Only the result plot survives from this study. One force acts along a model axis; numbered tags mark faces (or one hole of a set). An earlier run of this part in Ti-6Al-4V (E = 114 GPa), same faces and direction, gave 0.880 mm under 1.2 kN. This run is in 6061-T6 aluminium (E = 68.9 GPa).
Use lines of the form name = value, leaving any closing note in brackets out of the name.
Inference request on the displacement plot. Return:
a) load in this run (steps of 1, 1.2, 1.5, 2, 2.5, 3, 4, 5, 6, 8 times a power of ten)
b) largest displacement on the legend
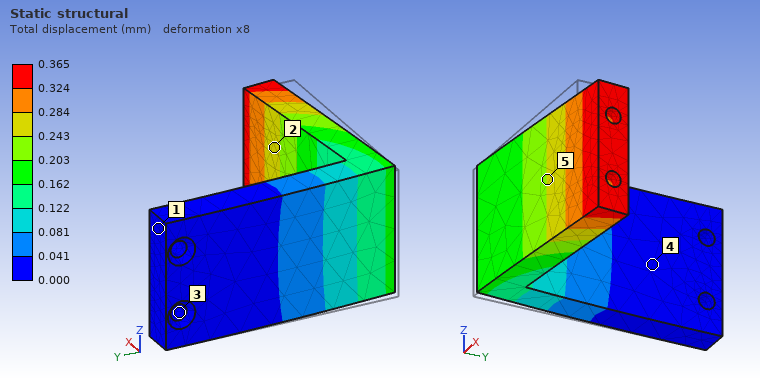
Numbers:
load in this run = 300 N
largest displacement on the legend = 0.365 mm
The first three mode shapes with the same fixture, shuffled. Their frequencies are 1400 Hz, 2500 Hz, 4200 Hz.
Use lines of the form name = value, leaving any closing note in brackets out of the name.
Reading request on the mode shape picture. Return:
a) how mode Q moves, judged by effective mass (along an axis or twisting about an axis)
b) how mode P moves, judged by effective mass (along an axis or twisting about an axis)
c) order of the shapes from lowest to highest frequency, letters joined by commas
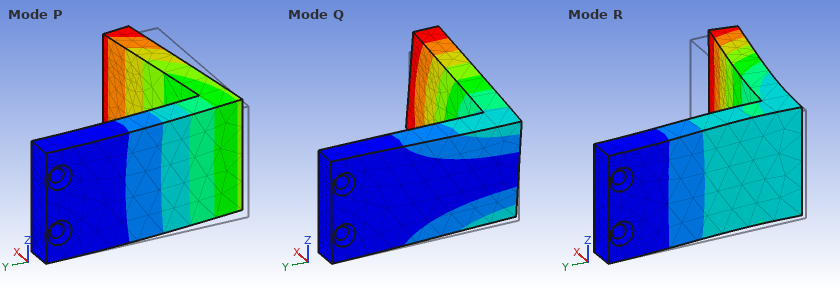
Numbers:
how mode Q moves, judged by effective mass = along Z
how mode P moves, judged by effective mass = along X
order of the shapes from lowest to highest frequency, letters joined by commas = P, Q, R
